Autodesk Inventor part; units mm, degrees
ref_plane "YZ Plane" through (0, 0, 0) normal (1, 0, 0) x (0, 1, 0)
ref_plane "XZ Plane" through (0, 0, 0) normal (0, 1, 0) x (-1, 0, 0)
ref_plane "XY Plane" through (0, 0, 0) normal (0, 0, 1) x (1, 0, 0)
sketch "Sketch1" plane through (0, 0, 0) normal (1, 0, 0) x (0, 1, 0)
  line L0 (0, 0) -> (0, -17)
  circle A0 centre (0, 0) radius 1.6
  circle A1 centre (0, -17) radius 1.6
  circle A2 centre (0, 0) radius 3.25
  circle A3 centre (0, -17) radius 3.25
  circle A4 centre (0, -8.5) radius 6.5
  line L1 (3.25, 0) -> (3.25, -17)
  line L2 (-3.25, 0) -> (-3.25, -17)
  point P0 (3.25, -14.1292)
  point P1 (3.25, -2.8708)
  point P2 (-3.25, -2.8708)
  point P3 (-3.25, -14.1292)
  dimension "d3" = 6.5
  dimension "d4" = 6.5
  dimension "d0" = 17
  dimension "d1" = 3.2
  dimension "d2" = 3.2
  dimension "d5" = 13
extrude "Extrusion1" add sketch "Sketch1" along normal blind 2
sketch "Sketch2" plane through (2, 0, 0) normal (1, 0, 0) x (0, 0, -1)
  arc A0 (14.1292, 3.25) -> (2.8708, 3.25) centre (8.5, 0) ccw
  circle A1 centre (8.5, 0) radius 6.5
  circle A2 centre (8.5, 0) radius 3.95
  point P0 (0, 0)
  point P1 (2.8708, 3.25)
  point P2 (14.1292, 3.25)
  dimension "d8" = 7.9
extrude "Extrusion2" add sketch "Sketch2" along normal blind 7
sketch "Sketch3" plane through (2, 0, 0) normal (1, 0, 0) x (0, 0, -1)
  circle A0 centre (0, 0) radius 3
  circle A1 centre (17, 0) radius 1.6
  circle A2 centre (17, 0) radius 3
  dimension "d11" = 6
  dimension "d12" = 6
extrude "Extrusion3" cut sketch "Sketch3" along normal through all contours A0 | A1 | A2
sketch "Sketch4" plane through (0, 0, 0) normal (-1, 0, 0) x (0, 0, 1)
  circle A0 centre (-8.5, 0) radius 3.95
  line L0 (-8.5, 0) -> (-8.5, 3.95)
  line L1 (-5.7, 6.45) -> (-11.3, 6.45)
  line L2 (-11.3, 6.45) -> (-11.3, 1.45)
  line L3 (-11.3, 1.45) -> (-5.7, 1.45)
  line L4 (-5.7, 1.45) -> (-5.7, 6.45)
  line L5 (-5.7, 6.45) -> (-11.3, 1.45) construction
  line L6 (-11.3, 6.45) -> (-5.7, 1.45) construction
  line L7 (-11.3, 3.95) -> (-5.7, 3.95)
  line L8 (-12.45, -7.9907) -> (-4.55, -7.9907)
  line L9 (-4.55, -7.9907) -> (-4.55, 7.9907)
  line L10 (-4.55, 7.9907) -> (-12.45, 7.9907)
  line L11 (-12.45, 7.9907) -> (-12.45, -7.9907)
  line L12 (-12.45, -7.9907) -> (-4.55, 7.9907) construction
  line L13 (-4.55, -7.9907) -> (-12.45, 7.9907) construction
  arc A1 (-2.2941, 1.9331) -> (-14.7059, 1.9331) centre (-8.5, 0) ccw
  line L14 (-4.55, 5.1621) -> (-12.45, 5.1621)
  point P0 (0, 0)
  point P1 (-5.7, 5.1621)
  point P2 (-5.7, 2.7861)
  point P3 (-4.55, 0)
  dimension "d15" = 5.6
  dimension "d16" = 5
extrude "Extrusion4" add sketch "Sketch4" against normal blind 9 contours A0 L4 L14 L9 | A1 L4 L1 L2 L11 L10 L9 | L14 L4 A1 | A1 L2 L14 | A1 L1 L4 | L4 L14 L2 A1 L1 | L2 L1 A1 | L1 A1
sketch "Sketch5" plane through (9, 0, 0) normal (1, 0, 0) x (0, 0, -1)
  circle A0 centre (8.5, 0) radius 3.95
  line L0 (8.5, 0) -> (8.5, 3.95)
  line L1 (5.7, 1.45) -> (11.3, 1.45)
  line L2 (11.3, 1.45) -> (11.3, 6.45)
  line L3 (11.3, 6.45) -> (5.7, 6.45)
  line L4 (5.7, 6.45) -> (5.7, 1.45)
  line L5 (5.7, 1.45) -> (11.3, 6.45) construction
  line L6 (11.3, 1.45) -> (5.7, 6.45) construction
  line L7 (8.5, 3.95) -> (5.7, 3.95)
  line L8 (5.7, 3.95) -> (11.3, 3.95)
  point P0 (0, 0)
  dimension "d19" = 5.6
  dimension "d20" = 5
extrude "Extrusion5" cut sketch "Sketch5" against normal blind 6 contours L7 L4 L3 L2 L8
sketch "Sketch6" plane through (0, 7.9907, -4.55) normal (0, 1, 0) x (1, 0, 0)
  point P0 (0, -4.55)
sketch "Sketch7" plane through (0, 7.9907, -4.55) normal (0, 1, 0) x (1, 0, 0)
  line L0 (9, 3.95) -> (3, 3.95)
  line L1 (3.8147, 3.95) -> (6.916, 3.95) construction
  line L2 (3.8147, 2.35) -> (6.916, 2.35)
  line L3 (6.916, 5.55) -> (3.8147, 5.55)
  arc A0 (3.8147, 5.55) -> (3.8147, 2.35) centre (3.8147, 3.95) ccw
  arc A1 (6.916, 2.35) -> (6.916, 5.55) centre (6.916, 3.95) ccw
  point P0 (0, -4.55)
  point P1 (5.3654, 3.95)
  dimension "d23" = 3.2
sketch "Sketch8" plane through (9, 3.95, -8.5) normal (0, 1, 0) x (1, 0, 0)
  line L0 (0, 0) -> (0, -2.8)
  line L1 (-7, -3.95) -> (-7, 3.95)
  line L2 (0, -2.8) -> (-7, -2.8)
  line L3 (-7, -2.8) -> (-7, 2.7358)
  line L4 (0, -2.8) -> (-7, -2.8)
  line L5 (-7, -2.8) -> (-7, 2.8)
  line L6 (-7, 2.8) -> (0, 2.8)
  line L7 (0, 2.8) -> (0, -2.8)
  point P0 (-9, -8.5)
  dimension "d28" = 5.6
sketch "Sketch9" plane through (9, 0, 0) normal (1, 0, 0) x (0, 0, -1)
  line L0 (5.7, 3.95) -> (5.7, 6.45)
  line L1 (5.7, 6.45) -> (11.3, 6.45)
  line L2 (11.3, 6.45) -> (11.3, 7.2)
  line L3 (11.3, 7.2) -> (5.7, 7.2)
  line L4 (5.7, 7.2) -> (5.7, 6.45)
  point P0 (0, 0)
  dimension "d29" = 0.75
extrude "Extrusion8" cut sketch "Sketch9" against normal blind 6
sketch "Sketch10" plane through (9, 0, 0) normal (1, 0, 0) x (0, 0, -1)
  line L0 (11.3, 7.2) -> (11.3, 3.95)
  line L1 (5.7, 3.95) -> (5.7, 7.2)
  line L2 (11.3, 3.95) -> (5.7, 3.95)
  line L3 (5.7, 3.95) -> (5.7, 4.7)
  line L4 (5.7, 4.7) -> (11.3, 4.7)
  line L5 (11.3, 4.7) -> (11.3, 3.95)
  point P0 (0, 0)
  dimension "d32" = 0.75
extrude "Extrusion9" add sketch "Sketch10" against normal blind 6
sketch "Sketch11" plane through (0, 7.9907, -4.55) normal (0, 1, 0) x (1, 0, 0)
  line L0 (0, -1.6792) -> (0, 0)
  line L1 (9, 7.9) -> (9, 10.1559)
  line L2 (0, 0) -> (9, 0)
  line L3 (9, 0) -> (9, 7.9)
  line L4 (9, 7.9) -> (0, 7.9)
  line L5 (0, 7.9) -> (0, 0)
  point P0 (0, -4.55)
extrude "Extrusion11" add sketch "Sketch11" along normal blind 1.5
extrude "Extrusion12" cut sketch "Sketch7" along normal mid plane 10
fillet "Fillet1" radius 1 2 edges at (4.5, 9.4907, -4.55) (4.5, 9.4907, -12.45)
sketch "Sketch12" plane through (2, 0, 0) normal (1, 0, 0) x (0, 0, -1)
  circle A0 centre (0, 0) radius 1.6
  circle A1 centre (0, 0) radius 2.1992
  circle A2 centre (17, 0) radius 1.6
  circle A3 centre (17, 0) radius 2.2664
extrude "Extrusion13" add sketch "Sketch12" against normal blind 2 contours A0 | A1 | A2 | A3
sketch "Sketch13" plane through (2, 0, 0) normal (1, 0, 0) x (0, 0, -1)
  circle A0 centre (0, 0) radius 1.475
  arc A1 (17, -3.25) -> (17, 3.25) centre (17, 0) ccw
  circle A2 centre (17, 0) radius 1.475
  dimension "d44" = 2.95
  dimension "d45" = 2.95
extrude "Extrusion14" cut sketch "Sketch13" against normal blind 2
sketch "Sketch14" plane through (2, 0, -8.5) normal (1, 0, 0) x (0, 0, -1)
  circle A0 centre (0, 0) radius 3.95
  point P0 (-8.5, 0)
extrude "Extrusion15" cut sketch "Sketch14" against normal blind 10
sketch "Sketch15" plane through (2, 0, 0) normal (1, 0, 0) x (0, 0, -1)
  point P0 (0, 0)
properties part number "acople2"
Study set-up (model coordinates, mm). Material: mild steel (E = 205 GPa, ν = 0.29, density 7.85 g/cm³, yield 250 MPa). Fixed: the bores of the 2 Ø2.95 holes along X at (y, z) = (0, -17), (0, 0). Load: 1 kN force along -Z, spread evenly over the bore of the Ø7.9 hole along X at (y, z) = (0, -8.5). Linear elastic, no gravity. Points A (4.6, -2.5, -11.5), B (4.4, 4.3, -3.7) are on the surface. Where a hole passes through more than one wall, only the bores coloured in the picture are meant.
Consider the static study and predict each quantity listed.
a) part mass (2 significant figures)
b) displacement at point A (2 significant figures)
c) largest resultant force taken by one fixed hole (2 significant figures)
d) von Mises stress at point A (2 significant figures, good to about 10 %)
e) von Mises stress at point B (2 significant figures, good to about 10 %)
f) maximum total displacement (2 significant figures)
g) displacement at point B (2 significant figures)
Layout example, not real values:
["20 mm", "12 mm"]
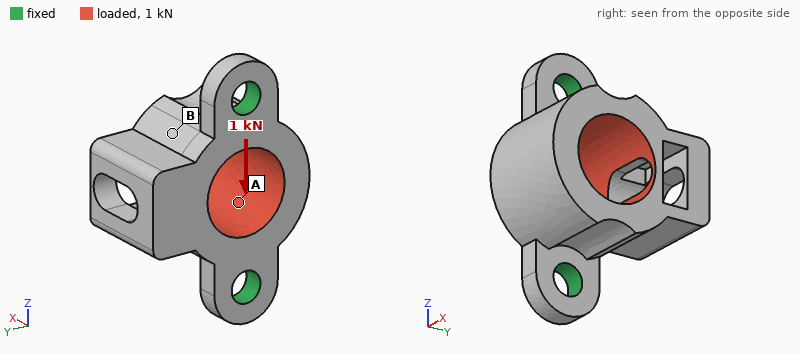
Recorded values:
["7.1 g", "2.3 µm", "560 N", "37 MPa", "15 MPa", "4.4 µm", "2.0 µm"]
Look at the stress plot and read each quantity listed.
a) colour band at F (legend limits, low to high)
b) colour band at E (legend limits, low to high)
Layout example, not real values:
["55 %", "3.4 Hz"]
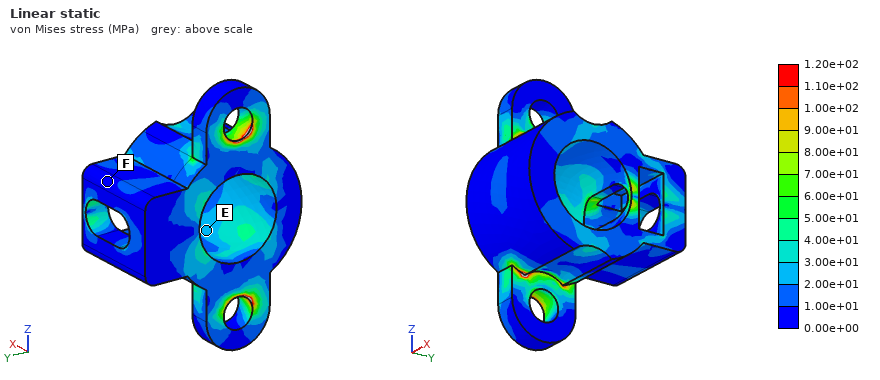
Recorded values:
["0.00e+00 to 1.00e+01 MPa", "2.00e+01 to 3.00e+01 MPa"]
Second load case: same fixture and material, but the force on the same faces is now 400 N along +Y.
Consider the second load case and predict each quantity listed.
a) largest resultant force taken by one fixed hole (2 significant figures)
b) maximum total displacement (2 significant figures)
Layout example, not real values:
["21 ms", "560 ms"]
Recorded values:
["200 N", "13 µm"]
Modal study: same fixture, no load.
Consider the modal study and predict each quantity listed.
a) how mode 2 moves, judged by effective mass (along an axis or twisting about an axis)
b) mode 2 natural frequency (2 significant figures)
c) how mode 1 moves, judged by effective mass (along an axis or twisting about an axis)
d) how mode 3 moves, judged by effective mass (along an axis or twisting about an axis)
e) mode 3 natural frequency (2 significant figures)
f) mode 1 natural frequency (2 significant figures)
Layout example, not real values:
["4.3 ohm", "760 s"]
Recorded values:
["along X", "31 kHz", "along Y", "along Z", "33 kHz", "11 kHz"]
